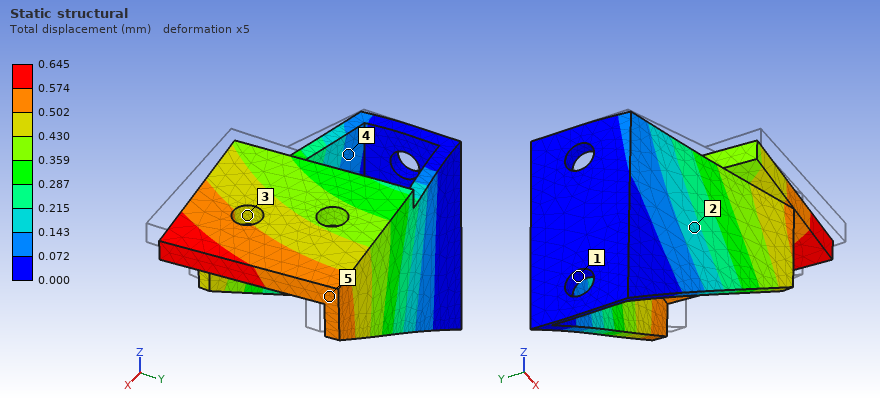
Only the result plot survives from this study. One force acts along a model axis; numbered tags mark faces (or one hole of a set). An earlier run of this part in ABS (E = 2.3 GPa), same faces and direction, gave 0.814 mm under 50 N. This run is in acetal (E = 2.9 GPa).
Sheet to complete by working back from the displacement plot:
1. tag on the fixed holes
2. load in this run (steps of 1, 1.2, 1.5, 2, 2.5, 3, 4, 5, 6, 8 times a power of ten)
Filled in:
1
50 N
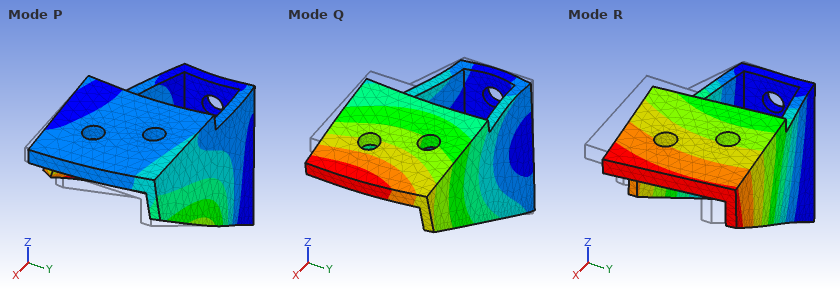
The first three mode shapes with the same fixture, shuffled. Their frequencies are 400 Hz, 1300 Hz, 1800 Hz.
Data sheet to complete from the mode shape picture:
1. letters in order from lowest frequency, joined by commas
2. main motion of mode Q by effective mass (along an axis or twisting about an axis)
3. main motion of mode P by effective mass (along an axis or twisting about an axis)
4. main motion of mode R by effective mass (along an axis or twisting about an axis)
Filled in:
R, Q, P
along Z
along X
along Y
